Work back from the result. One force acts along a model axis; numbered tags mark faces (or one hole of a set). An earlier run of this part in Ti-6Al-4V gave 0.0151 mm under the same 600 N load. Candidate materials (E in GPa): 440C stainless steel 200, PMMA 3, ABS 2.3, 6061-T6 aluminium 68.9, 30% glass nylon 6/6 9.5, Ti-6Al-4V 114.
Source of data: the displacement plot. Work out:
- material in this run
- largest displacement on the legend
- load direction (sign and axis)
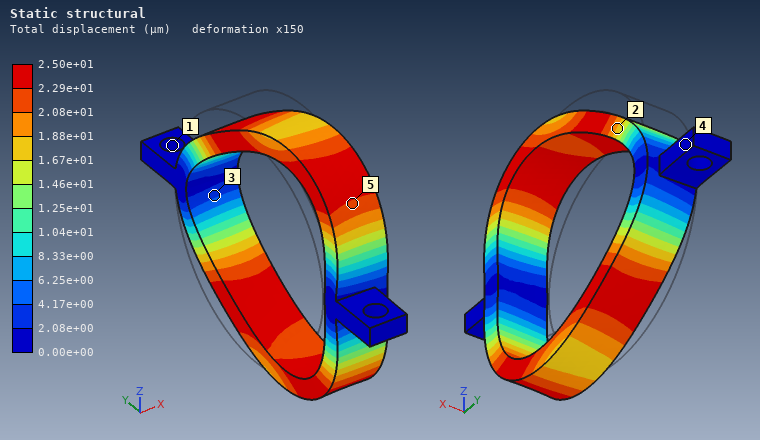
6061-T6 aluminium
2.50e+01 µm
-Y
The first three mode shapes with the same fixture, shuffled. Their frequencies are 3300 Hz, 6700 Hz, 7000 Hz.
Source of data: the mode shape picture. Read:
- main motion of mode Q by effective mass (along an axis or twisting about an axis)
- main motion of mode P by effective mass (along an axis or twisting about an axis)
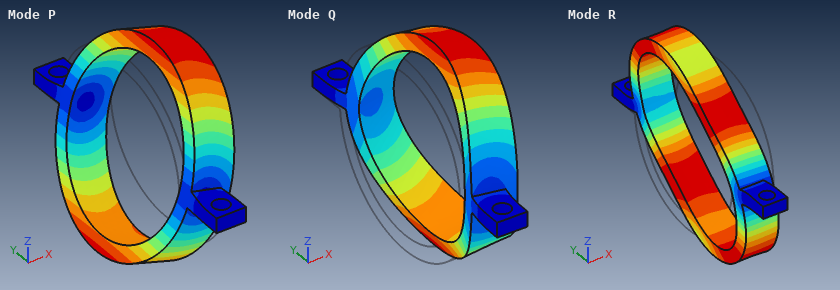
along X
twisting about Y
